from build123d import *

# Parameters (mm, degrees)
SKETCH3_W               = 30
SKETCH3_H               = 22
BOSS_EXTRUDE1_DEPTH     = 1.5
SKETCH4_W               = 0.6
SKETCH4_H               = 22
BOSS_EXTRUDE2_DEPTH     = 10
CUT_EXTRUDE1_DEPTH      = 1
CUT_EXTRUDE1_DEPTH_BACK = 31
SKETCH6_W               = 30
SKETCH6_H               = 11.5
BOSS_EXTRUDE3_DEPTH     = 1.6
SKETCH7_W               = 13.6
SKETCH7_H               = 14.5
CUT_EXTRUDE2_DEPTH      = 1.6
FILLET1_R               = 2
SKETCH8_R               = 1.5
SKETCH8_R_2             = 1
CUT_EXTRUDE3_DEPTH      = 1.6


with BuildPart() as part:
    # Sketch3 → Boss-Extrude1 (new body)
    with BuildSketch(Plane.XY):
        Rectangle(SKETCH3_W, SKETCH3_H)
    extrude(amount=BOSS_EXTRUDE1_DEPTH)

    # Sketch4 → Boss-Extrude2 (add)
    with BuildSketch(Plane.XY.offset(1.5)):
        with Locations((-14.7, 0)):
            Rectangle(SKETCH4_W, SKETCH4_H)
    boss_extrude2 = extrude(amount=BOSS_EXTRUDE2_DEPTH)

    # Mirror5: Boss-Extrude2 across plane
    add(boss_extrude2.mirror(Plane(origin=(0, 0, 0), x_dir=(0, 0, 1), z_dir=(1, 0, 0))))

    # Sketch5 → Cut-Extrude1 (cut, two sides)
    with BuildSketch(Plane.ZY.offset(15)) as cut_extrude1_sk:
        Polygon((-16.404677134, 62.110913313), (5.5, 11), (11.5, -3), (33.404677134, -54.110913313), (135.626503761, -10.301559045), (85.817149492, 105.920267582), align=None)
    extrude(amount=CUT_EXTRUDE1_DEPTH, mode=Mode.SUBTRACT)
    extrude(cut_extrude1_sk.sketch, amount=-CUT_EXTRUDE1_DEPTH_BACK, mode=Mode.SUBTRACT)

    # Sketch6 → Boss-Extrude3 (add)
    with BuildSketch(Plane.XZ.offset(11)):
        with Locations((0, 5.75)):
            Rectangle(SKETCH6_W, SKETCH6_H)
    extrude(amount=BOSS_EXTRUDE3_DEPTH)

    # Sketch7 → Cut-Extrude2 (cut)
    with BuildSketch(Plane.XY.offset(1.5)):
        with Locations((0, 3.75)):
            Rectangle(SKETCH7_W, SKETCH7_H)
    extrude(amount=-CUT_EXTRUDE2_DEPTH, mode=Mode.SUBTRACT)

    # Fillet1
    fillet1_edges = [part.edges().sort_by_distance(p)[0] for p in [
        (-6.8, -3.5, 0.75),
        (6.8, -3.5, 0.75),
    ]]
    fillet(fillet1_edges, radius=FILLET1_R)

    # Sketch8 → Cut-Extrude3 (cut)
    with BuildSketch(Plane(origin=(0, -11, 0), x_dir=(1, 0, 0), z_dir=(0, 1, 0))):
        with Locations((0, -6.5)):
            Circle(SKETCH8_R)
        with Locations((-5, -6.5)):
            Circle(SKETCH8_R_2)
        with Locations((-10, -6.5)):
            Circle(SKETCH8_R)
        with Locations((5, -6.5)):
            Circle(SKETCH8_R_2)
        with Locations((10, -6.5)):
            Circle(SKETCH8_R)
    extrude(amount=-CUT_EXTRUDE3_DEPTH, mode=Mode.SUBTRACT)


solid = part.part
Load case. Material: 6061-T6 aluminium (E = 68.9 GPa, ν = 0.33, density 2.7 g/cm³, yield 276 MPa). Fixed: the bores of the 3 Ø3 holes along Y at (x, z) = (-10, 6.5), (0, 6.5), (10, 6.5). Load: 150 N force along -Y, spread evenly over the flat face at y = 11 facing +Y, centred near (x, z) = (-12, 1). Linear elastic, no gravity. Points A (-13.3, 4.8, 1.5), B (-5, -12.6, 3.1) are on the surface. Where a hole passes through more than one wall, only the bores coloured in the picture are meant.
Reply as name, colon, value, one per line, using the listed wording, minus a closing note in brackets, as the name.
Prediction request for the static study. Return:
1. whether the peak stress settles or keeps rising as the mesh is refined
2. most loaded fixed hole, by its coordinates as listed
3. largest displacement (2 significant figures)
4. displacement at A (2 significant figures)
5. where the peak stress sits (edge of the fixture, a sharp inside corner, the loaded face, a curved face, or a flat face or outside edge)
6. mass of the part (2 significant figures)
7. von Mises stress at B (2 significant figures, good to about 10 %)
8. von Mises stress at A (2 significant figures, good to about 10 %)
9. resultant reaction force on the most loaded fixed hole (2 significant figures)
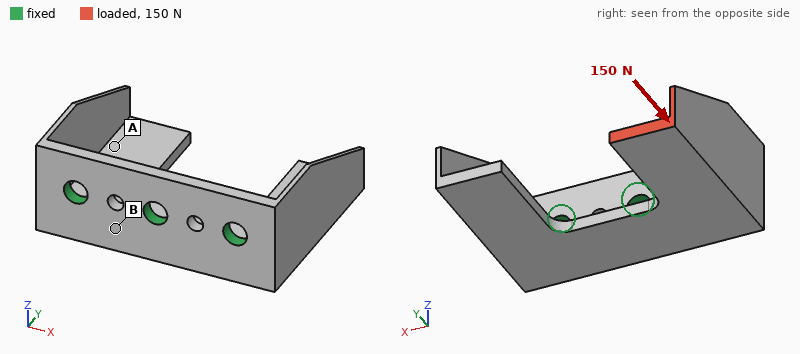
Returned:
whether the peak stress settles or keeps rising as the mesh is refined: keeps rising
most loaded fixed hole, by its coordinates as listed: (-10, 6.5)
largest displacement: 76 µm
displacement at A: 54 µm
where the peak stress sits: edge of the fixture
mass of the part: 3.8 g
von Mises stress at B: 24 MPa
von Mises stress at A: 9.6 MPa
resultant reaction force on the most loaded fixed hole: 130 N
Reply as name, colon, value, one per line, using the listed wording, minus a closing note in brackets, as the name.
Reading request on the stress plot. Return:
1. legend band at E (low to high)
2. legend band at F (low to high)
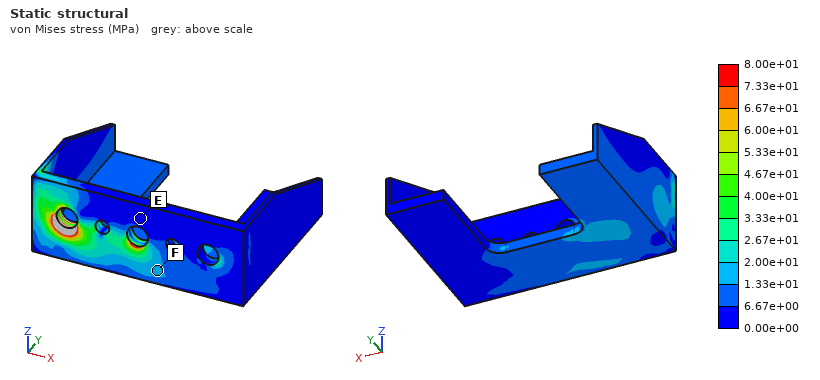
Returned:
legend band at E: 0.00e+00 to 6.67e+00 MPa
legend band at F: 1.33e+01 to 2.00e+01 MPa
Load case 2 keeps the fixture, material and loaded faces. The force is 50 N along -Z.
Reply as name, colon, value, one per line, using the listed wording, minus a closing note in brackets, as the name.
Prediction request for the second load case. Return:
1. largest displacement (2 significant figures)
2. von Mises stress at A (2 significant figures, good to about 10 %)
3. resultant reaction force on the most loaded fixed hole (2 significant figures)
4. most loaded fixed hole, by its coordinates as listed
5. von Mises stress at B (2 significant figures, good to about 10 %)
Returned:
largest displacement: 0.24 mm
von Mises stress at A: 49 MPa
resultant reaction force on the most loaded fixed hole: 62 N
most loaded fixed hole, by its coordinates as listed: (-10, 6.5)
von Mises stress at B: 42 MPa
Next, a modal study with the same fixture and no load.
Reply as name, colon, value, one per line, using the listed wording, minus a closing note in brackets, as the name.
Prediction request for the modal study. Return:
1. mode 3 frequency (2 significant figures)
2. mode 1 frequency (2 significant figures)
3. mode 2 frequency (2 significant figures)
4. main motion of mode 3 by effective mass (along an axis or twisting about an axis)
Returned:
mode 3 frequency: 7600 Hz
mode 1 frequency: 4300 Hz
mode 2 frequency: 4400 Hz
main motion of mode 3 by effective mass: along X
